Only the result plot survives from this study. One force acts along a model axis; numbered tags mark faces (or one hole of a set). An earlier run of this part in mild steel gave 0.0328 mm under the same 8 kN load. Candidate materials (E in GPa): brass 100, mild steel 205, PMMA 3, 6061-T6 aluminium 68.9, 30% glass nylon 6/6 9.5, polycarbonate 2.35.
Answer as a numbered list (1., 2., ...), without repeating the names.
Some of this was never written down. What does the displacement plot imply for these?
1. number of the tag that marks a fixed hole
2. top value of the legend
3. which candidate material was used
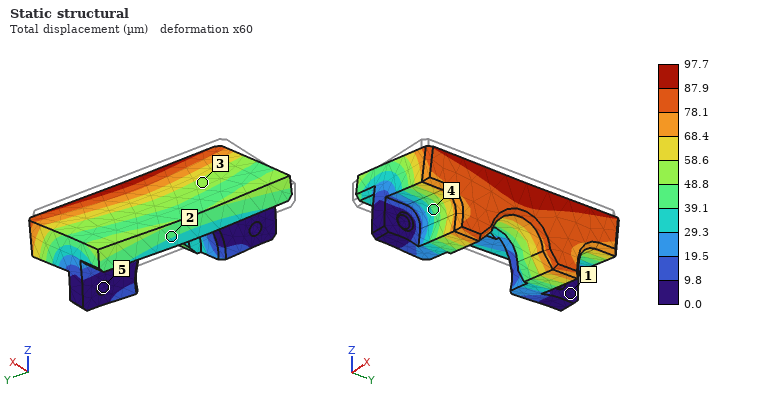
1. 5
2. 97.7 µm
3. 6061-T6 aluminium
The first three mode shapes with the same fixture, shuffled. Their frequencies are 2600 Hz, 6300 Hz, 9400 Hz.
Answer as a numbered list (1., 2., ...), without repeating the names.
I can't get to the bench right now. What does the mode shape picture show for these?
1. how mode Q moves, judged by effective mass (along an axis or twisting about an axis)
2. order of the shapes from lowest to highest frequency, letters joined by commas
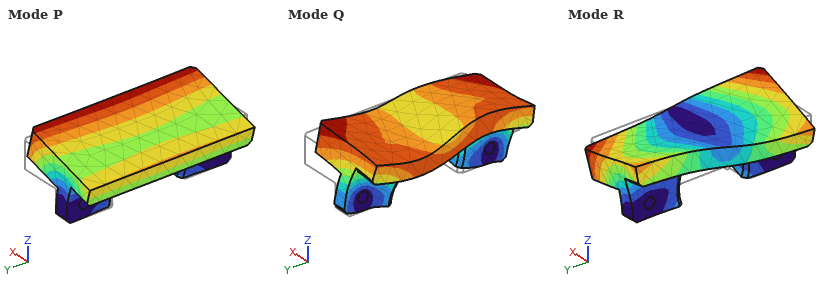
1. along Y
2. P, R, Q
